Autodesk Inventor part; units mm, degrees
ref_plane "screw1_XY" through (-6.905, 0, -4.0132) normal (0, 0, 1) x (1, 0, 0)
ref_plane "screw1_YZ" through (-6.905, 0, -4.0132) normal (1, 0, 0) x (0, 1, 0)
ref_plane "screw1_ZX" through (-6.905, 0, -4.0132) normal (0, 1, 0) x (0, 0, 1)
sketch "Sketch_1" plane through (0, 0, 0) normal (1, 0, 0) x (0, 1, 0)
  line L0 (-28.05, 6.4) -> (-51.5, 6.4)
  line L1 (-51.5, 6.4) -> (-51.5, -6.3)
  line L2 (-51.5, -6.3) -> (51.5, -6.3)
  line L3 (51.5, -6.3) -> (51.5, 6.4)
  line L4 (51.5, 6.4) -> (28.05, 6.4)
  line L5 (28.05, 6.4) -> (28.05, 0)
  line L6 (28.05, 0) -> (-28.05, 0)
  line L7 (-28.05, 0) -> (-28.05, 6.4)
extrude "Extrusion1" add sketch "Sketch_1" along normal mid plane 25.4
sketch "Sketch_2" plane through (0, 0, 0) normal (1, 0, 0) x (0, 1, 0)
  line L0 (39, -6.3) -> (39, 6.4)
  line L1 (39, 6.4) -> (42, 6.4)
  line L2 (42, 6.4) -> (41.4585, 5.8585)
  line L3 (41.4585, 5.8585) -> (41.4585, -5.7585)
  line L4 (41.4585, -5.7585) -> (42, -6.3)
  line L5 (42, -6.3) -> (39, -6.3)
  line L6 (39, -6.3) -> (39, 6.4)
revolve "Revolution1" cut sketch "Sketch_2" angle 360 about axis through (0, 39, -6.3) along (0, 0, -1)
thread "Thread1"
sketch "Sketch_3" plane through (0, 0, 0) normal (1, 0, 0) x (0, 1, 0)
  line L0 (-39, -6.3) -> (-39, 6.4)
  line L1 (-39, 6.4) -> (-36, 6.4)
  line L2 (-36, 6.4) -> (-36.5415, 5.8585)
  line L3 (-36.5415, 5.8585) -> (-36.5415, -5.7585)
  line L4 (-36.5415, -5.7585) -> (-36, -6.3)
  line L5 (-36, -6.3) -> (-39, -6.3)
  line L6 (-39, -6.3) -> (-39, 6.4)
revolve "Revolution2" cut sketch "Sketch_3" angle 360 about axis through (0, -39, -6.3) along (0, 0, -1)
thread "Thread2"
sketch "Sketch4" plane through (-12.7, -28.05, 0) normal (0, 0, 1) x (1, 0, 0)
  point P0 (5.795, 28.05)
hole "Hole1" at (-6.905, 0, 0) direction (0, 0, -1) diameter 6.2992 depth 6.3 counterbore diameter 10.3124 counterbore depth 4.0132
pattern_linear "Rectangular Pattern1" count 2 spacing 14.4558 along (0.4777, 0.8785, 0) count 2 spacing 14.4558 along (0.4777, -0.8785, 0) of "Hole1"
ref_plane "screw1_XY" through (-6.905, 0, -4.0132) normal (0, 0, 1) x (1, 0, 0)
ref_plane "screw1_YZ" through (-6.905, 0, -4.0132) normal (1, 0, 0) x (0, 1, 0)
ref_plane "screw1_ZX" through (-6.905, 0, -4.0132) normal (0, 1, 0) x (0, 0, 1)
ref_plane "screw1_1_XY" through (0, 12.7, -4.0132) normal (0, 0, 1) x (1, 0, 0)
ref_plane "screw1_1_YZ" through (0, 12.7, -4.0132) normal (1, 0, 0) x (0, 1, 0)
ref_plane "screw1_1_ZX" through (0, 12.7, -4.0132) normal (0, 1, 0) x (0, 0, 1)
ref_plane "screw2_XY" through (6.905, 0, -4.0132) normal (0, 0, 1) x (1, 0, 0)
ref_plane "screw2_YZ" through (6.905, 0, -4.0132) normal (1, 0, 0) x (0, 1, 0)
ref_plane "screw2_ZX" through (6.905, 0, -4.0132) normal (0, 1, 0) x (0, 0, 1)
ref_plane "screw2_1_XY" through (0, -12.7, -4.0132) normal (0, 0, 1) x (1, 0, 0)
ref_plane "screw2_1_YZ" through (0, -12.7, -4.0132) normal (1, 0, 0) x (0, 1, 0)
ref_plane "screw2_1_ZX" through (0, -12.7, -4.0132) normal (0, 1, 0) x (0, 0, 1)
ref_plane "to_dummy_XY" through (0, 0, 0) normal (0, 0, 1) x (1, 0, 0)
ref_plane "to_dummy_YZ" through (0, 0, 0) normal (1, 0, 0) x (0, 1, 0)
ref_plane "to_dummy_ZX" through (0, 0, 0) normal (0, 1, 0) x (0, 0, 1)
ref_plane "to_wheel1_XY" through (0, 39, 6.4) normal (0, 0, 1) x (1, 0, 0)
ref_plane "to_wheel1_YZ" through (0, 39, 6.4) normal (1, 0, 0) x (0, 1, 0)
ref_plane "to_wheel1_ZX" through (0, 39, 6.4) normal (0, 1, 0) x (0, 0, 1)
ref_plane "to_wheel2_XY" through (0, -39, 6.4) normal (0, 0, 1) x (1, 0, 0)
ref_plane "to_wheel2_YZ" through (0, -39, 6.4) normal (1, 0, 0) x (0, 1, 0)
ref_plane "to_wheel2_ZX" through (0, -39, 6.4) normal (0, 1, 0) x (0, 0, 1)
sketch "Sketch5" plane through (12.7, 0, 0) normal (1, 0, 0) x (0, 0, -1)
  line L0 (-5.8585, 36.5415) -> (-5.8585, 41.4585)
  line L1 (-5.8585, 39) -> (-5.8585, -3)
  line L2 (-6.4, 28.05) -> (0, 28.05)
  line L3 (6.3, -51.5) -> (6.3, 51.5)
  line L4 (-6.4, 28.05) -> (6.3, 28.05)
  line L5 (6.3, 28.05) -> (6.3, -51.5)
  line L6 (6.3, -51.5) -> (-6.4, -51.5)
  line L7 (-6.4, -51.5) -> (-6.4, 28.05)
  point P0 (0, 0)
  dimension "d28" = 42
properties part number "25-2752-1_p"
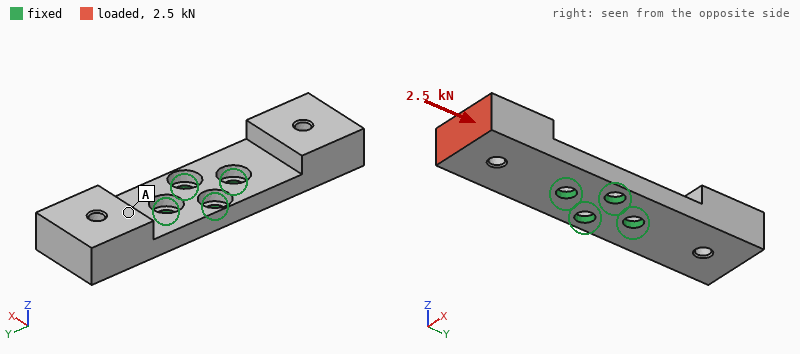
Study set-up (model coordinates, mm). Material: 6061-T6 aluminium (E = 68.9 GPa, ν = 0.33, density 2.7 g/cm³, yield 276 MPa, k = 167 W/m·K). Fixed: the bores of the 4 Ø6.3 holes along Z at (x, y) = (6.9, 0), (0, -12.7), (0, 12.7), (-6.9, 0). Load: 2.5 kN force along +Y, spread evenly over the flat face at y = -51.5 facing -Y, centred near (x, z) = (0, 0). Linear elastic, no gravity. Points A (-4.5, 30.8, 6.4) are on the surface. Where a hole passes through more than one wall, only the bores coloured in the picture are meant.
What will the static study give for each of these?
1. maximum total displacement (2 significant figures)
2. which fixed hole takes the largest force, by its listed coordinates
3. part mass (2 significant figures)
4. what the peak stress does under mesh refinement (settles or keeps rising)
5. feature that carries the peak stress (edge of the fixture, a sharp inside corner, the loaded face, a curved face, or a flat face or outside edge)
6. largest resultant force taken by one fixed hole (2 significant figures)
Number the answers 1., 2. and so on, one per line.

1. 0.20 mm
2. (0, -12.7)
3. 59 g
4. keeps rising
5. edge of the fixture
6. 1.1 kN
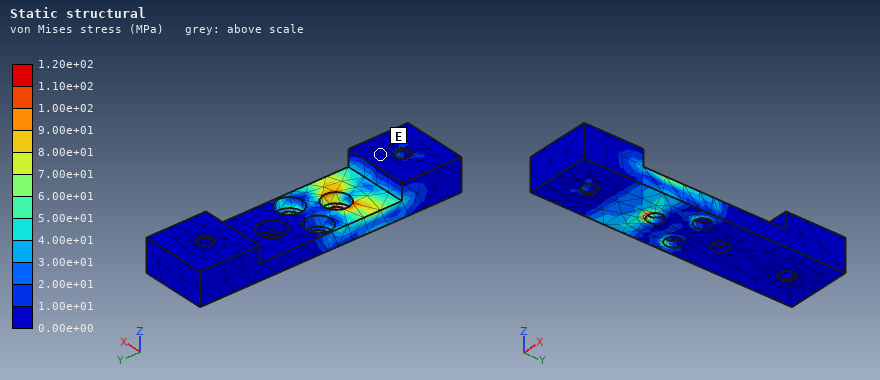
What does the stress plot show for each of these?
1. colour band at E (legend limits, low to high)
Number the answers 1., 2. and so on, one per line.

1. 0.00e+00 to 1.00e+01 MPa
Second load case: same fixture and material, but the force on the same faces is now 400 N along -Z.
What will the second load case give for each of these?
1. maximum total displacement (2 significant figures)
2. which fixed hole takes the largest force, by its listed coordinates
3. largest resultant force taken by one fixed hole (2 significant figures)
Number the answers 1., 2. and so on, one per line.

1. 0.27 mm
2. (0, -12.7)
3. 1.8 kN
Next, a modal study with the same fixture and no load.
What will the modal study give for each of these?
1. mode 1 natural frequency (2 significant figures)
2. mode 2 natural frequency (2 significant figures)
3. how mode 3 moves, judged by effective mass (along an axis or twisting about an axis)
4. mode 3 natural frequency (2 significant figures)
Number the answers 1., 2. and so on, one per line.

1. 2000 Hz
2. 2000 Hz
3. twisting about Z
4. 4800 Hz
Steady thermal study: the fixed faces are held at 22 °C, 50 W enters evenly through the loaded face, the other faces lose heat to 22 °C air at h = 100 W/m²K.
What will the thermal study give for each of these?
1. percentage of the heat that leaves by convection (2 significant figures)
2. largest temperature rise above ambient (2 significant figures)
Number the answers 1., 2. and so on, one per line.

1. 22 %
2. 54 K
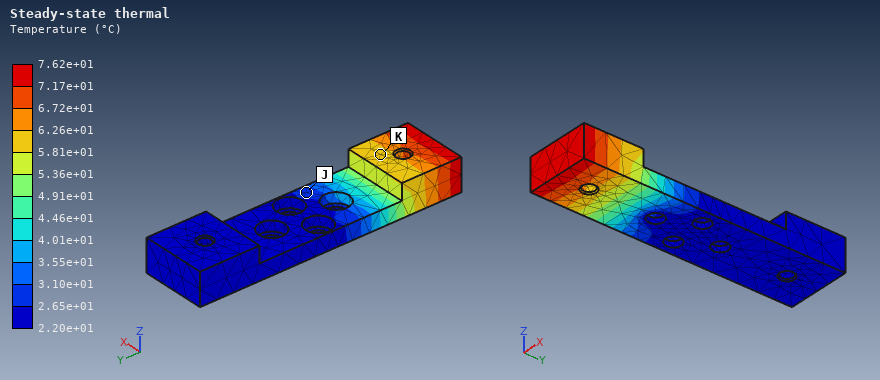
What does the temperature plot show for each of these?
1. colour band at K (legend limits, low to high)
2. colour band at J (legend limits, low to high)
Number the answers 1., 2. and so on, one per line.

1. 5.81e+01 to 6.26e+01 °C
2. 2.65e+01 to 3.10e+01 °C
